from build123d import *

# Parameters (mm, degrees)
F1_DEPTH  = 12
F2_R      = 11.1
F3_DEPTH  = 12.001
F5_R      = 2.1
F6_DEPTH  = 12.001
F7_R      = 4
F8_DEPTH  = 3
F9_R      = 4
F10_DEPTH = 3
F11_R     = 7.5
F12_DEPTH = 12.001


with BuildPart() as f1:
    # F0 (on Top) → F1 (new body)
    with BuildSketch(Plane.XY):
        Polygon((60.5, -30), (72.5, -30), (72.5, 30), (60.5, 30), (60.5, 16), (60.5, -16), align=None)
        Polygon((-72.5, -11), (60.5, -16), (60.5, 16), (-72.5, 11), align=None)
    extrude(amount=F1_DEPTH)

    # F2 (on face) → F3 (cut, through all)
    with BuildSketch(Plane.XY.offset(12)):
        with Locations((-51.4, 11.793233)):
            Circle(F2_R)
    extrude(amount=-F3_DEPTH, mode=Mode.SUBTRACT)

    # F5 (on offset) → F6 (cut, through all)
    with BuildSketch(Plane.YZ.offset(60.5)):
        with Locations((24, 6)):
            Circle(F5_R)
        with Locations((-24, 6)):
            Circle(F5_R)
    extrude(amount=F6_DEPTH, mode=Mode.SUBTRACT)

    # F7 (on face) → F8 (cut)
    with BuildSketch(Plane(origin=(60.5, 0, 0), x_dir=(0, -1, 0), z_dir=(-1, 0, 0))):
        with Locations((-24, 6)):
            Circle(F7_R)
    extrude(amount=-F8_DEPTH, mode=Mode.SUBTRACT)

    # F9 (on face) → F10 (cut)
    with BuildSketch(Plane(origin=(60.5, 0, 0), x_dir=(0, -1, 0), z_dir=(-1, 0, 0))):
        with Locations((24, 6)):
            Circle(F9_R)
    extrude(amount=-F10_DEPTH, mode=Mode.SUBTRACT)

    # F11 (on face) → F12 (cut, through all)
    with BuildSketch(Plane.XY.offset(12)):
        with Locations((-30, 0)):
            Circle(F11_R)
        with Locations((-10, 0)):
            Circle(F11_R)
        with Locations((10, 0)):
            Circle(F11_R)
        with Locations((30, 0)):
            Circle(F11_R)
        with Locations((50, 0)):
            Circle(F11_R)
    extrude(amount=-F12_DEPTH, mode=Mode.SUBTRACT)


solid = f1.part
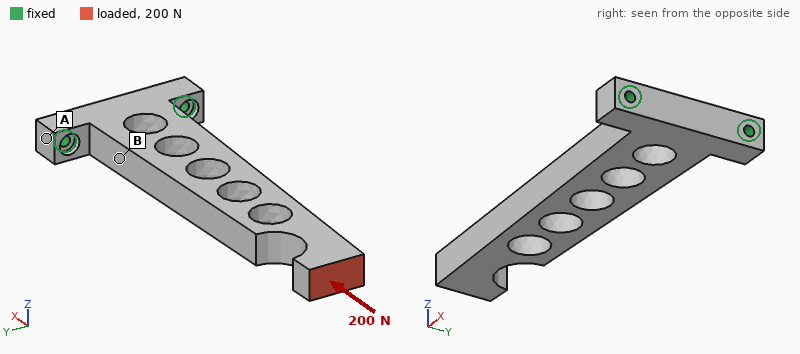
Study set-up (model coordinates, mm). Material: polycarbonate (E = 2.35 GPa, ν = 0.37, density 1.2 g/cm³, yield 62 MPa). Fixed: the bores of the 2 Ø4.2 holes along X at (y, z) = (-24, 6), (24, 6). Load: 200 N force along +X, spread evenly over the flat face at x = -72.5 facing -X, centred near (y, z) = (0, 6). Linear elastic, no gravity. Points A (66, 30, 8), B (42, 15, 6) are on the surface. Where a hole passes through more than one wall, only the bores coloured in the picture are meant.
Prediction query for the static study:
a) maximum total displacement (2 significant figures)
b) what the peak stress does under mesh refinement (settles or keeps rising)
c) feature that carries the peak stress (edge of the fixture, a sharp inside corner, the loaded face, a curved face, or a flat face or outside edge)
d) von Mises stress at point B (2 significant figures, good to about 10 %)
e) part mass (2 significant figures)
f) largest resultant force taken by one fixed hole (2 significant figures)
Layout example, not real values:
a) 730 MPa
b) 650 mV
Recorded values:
a) 0.22 mm
b) keeps rising
c) edge of the fixture
d) 0.95 MPa
e) 46 g
f) 110 N
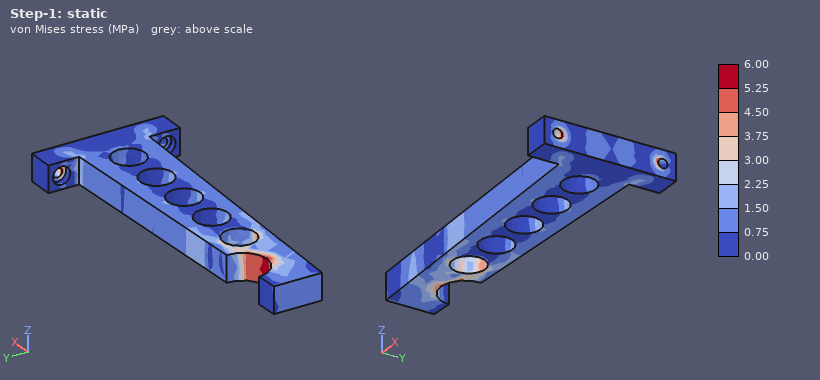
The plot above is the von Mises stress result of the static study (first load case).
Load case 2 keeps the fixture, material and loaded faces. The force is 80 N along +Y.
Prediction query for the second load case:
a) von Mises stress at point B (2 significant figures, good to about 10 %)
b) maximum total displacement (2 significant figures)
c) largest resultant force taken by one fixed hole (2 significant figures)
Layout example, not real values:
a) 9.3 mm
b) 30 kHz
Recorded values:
a) 5.5 MPa
b) 1.8 mm
c) 280 N
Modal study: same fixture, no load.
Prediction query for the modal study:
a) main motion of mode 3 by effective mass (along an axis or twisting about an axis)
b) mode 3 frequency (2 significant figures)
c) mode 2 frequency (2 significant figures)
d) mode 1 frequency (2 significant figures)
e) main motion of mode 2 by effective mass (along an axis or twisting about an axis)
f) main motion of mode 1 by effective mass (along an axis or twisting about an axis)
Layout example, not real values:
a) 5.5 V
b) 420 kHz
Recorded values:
a) along Z
b) 650 Hz
c) 370 Hz
d) 120 Hz
e) along Y
f) along Z
